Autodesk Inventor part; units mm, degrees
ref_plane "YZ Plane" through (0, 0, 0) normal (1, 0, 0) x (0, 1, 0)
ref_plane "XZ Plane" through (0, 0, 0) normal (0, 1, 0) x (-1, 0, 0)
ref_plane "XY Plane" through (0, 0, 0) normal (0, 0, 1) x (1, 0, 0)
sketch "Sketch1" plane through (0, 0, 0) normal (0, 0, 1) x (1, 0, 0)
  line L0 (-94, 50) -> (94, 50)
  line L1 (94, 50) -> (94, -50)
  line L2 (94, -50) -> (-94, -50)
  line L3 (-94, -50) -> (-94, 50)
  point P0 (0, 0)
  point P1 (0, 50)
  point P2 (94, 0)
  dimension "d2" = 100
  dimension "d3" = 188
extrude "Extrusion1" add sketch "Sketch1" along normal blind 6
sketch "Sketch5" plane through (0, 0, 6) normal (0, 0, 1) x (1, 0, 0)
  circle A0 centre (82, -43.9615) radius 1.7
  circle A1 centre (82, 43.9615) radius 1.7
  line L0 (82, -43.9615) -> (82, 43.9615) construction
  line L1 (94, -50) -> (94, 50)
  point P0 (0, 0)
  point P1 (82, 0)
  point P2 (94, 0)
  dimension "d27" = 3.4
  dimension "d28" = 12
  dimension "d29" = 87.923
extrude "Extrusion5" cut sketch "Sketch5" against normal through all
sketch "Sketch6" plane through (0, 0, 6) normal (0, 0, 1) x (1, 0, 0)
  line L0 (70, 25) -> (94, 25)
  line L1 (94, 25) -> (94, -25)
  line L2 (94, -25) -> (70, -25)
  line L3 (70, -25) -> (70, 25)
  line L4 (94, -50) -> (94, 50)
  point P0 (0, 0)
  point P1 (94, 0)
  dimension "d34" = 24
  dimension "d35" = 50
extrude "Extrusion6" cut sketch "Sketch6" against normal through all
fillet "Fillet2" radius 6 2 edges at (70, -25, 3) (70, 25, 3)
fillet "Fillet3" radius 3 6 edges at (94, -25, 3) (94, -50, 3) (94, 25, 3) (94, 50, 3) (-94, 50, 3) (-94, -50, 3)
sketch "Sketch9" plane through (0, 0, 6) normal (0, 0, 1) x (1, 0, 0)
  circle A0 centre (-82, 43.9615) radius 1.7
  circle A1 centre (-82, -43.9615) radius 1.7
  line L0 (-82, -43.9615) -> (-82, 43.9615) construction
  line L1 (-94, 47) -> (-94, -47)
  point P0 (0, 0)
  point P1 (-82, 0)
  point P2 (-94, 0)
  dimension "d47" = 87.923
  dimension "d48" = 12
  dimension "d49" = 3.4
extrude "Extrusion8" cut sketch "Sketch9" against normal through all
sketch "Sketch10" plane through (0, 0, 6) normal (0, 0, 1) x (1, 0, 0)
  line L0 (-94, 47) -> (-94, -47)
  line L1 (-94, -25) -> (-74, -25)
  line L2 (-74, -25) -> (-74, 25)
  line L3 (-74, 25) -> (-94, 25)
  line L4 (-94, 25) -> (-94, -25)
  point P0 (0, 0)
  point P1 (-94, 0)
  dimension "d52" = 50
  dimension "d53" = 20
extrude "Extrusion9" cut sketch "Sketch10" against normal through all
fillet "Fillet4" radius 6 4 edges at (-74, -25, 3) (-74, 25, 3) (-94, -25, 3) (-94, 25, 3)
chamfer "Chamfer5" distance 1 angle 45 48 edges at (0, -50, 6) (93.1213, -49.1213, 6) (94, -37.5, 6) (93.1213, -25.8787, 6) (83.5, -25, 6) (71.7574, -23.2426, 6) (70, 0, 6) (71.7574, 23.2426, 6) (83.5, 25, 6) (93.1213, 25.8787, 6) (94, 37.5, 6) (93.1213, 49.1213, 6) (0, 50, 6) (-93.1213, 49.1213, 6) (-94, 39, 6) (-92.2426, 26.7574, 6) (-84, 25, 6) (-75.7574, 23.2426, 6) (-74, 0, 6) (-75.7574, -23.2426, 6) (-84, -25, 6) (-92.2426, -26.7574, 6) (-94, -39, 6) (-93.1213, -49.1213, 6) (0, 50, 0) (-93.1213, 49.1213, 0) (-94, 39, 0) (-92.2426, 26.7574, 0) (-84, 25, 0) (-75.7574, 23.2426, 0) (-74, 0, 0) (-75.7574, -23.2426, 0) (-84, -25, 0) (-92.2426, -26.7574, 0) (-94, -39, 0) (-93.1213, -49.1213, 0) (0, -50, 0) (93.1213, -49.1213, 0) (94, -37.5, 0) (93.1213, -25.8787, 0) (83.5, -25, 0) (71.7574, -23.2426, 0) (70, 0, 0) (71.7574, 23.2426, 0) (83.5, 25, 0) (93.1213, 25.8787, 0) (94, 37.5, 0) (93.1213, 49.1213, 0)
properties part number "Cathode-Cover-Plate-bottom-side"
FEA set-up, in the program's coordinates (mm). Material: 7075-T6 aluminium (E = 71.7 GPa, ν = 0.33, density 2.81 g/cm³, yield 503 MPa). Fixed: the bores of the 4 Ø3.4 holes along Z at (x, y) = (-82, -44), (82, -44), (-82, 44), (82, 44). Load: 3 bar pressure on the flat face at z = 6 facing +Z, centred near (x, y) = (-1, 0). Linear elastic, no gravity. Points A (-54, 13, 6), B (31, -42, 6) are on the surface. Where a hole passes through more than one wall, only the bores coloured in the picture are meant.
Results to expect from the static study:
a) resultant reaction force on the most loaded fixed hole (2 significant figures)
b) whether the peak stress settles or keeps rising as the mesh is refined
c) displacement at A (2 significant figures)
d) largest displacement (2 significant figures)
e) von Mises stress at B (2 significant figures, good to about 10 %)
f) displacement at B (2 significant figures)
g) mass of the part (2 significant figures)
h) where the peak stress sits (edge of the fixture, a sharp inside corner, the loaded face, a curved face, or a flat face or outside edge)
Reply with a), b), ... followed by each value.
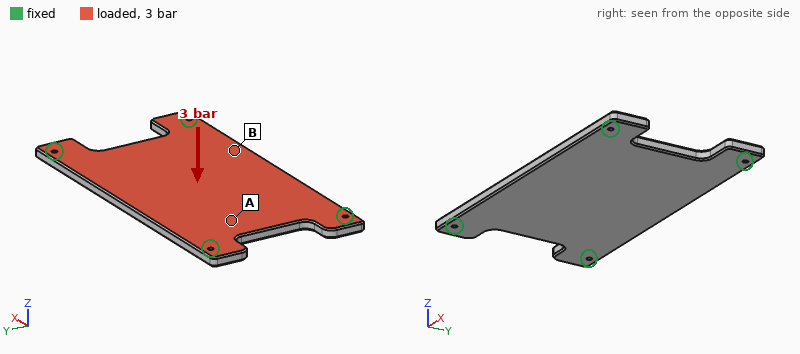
a) 1.2 kN
b) keeps rising
c) 0.34 mm
d) 0.73 mm
e) 57 MPa
f) 0.56 mm
g) 280 g
h) edge of the fixture
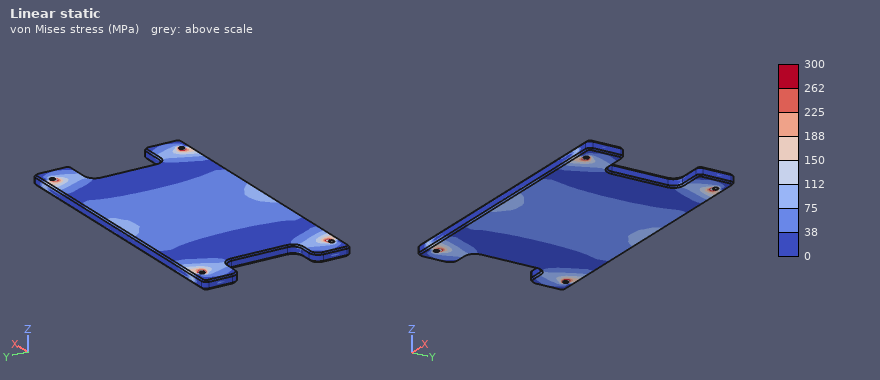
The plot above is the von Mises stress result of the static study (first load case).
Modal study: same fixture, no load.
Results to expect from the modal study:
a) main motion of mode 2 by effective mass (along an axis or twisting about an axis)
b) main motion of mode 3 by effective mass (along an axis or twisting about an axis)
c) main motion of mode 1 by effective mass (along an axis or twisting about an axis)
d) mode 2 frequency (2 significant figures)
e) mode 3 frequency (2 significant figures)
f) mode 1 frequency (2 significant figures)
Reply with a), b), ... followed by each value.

a) twisting about X
b) twisting about Y
c) along Z
d) 1600 Hz
e) 2400 Hz
f) 880 Hz
